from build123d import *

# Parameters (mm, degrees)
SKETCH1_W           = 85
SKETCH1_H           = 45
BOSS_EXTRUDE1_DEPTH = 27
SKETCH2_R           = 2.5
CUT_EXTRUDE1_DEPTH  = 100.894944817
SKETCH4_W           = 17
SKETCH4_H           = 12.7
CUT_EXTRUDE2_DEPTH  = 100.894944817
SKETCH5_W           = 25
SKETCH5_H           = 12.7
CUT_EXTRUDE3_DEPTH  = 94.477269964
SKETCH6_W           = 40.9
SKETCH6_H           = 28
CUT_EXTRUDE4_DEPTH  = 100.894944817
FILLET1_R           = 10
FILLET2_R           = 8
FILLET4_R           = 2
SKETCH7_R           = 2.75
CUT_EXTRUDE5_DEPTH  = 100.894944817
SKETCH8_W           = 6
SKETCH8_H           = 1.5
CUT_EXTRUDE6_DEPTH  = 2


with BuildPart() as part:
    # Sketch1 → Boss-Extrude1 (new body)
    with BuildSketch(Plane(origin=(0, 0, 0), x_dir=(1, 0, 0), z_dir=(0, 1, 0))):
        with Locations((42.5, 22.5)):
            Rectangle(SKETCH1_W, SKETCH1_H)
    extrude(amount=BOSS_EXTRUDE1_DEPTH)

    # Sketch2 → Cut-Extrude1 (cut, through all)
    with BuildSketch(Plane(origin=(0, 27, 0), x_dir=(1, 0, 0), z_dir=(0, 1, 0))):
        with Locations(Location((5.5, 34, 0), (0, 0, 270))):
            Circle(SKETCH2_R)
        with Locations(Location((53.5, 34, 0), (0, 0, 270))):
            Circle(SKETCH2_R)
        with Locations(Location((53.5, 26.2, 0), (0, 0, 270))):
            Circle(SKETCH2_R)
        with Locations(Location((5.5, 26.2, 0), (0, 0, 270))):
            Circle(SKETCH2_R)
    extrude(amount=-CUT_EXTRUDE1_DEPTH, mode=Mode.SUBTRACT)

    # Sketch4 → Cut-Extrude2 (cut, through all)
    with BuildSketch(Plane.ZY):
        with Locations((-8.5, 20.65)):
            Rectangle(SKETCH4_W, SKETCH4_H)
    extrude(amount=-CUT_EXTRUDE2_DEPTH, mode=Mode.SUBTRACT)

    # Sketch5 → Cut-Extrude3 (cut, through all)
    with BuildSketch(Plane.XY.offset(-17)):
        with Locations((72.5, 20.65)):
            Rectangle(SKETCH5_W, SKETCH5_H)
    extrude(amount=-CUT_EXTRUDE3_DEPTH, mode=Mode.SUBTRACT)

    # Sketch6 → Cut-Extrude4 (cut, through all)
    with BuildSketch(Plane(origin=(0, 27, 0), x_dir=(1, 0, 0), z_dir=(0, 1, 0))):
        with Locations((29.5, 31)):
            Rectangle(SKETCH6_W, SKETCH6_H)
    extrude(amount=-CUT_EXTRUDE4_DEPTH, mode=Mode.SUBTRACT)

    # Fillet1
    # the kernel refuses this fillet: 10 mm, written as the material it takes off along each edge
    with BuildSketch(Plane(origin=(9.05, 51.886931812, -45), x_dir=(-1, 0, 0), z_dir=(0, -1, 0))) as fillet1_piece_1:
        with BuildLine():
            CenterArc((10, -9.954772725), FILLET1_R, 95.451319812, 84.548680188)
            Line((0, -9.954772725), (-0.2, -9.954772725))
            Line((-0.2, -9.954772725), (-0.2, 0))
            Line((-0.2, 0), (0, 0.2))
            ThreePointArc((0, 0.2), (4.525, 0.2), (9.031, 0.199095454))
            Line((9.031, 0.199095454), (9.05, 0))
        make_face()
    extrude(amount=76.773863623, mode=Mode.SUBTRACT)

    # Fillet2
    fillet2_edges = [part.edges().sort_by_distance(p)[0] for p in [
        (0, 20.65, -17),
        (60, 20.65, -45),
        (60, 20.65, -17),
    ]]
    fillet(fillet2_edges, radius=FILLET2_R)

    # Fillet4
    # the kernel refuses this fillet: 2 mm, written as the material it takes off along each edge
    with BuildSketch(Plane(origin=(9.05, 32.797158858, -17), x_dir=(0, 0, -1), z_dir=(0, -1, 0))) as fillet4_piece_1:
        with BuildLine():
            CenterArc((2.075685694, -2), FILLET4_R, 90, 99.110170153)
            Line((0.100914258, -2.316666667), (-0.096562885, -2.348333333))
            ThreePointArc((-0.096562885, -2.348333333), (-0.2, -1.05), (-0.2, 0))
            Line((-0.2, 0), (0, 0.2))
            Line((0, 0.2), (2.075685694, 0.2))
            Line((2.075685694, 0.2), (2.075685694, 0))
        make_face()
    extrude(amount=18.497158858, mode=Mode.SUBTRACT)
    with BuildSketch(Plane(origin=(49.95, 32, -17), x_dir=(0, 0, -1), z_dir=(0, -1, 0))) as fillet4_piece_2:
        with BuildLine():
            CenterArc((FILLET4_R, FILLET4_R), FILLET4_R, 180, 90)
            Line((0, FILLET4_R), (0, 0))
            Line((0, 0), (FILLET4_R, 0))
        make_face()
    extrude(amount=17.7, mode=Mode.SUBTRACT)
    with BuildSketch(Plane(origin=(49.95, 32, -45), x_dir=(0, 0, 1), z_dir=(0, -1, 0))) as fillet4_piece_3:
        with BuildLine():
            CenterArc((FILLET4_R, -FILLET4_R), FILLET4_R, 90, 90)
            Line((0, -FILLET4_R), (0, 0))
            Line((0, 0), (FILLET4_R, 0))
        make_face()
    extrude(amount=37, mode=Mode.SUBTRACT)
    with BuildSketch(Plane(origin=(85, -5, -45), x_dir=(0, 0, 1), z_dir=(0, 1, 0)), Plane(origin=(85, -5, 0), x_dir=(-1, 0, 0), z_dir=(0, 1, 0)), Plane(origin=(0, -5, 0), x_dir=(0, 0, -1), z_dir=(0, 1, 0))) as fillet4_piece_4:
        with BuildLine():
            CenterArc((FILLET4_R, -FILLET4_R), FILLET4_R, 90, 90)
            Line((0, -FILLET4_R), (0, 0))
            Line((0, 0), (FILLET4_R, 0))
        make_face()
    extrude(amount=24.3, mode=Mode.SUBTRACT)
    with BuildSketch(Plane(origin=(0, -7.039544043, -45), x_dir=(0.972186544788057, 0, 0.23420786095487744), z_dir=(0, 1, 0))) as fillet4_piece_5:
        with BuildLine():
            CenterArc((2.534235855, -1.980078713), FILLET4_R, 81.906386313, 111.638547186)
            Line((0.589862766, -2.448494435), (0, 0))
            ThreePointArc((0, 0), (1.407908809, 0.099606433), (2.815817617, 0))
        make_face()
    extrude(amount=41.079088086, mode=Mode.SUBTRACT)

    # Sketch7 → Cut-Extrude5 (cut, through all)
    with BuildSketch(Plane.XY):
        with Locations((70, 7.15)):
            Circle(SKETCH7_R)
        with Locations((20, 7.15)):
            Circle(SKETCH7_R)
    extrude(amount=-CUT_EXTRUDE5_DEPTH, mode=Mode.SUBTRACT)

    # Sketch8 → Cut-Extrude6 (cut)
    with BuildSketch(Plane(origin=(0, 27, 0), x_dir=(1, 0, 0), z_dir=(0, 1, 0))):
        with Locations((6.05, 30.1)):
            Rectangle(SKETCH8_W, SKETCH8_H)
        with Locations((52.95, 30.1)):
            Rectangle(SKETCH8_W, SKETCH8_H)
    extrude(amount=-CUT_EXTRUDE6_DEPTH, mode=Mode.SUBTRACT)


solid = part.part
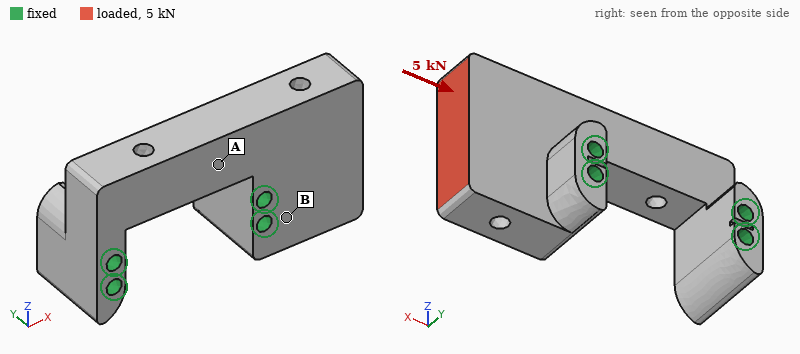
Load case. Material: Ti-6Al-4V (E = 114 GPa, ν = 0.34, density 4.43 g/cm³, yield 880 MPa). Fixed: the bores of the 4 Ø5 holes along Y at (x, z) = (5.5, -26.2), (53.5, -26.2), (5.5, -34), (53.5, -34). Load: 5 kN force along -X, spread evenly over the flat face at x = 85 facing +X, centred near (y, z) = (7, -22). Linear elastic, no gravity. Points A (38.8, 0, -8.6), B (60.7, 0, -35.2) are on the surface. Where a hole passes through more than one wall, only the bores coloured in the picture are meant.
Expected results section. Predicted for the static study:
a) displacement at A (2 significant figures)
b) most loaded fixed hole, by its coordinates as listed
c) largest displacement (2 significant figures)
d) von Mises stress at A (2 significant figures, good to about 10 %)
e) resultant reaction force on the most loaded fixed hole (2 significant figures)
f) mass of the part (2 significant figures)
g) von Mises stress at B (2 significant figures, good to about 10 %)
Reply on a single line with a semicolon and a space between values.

3.5 µm; (53.5, -26.2); 7.9 µm; 4.7 MPa; 3.4 kN; 180 g; 11 MPa
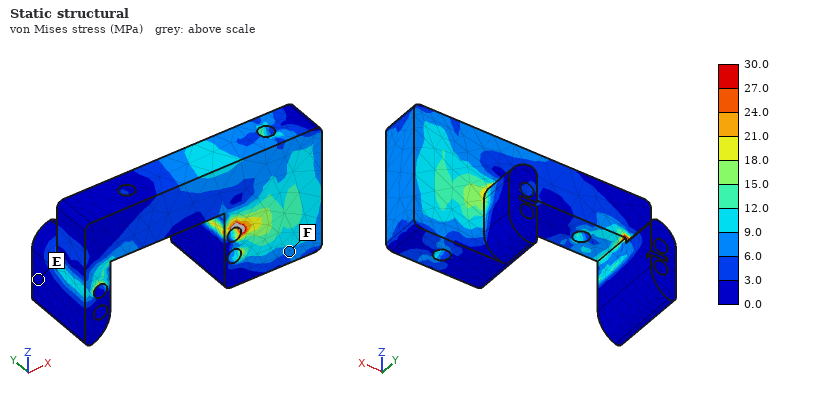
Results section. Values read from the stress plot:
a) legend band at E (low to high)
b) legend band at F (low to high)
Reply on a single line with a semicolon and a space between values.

0.0 to 3.0 MPa; 6.0 to 9.0 MPa
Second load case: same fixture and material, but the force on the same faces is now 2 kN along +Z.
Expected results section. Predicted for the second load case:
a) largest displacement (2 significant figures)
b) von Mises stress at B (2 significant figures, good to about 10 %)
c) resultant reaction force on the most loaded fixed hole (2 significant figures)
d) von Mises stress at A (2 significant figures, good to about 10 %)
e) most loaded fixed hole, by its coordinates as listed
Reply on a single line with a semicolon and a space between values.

13 µm; 14 MPa; 3.0 kN; 5.1 MPa; (53.5, -34)
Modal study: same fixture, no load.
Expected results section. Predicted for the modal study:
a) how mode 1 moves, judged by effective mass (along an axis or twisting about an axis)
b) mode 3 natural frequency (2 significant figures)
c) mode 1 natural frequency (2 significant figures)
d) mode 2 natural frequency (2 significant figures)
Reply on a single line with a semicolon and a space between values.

along Y; 9900 Hz; 8900 Hz; 9800 Hz
